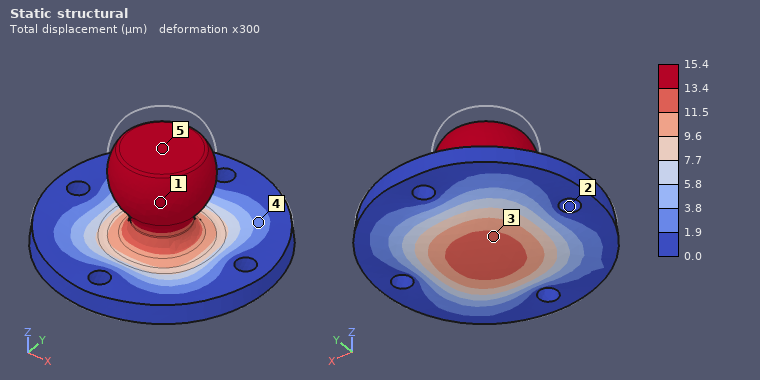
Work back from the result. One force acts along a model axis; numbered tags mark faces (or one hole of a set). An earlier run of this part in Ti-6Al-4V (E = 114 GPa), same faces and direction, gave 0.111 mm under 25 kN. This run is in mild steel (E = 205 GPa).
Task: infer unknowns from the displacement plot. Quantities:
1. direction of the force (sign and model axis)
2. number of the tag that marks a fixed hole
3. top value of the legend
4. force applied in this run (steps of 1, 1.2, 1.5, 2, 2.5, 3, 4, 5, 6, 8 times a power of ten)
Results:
-Z
2
15.4 µm
6 kN
